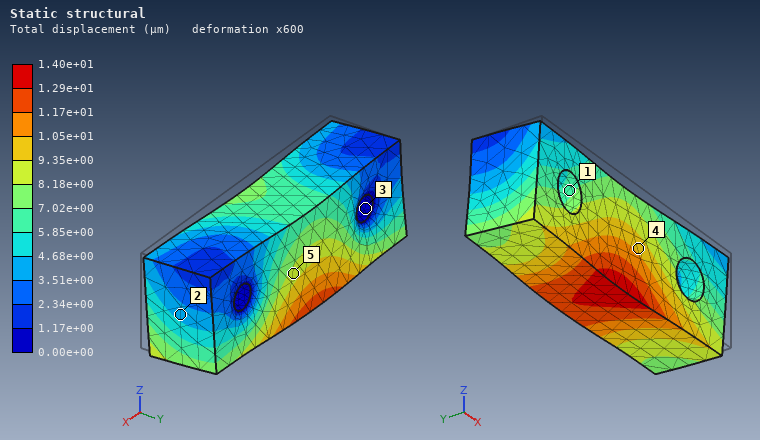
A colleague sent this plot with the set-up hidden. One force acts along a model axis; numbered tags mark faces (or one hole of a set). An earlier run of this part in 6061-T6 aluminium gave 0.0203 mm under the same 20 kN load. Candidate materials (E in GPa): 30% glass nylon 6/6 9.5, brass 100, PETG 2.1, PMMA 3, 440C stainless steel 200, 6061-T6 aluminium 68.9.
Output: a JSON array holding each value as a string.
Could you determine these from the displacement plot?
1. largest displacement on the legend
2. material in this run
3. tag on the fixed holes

["1.40e+01 µm", "brass", "3"]
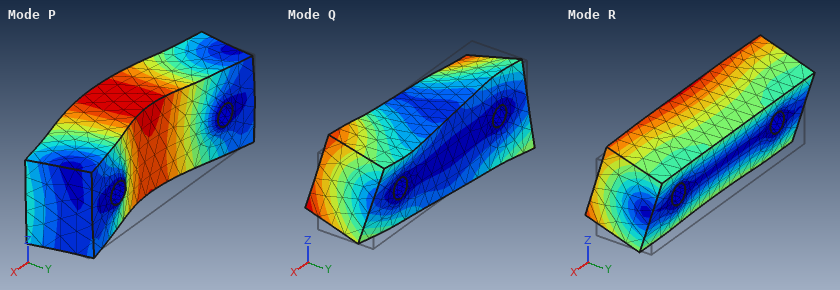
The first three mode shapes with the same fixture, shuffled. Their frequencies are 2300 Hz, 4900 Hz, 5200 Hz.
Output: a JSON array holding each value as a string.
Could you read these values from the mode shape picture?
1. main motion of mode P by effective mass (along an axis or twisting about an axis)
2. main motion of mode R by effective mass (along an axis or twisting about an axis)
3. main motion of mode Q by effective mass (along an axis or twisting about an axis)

["along Y", "along Z", "twisting about Y"]
